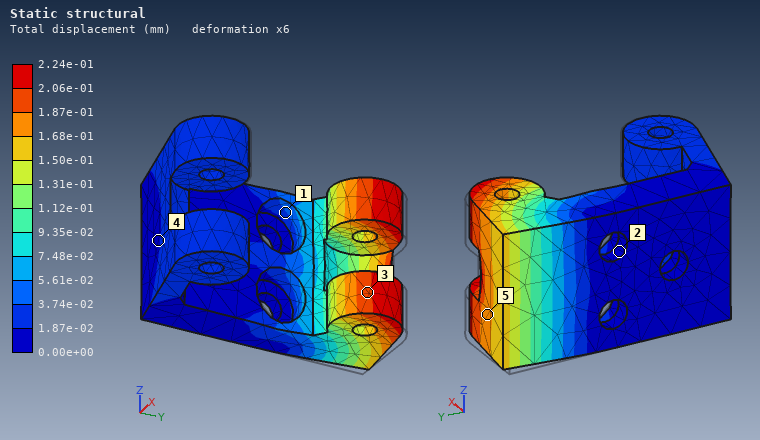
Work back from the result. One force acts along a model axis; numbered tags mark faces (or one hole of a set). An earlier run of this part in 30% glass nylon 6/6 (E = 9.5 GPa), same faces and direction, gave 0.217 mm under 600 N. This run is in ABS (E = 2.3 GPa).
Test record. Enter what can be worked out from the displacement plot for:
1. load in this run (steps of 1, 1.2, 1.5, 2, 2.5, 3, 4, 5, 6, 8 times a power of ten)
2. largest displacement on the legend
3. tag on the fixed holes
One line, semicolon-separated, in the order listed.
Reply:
150 N; 2.24e-01 mm; 2
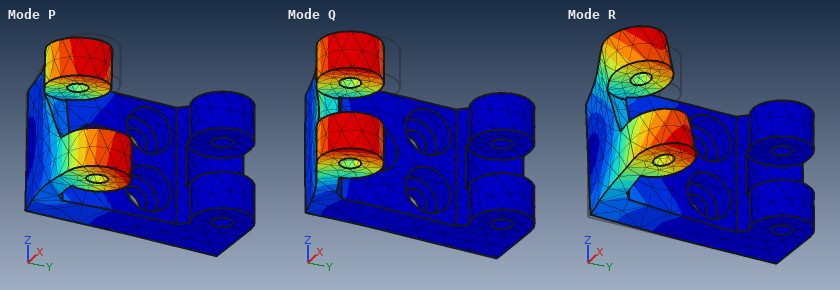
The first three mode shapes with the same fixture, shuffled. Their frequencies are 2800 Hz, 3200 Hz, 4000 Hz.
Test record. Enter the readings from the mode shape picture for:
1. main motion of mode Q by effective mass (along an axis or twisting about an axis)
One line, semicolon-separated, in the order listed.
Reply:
along Y
